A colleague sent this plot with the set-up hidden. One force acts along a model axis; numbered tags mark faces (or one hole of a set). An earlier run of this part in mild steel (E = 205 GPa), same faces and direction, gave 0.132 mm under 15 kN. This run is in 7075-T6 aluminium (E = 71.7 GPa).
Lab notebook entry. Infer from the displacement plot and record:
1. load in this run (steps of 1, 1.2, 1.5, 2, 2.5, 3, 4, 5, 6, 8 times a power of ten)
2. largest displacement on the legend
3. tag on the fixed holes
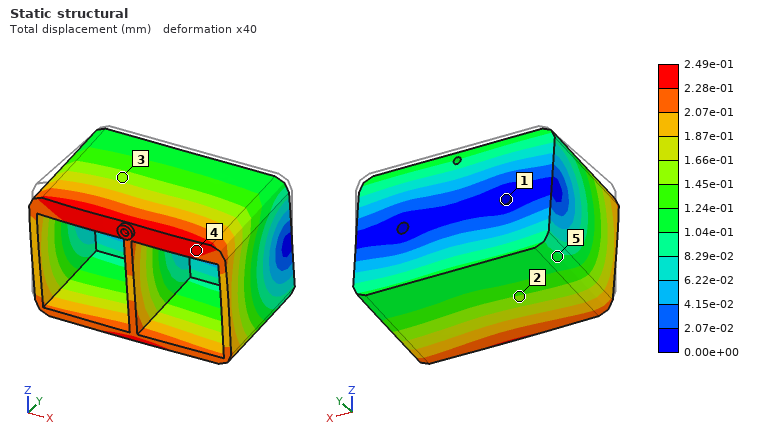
10 kN
2.49e-01 mm
1
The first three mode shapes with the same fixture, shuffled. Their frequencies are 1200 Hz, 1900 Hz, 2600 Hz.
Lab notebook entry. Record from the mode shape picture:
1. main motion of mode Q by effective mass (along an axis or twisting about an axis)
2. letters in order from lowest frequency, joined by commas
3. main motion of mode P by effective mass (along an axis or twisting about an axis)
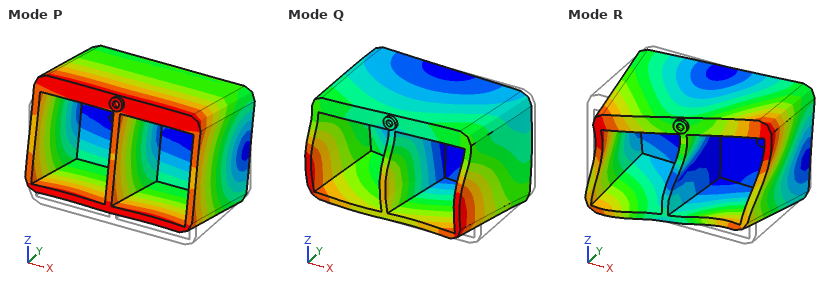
along X
P, R, Q
along Z
